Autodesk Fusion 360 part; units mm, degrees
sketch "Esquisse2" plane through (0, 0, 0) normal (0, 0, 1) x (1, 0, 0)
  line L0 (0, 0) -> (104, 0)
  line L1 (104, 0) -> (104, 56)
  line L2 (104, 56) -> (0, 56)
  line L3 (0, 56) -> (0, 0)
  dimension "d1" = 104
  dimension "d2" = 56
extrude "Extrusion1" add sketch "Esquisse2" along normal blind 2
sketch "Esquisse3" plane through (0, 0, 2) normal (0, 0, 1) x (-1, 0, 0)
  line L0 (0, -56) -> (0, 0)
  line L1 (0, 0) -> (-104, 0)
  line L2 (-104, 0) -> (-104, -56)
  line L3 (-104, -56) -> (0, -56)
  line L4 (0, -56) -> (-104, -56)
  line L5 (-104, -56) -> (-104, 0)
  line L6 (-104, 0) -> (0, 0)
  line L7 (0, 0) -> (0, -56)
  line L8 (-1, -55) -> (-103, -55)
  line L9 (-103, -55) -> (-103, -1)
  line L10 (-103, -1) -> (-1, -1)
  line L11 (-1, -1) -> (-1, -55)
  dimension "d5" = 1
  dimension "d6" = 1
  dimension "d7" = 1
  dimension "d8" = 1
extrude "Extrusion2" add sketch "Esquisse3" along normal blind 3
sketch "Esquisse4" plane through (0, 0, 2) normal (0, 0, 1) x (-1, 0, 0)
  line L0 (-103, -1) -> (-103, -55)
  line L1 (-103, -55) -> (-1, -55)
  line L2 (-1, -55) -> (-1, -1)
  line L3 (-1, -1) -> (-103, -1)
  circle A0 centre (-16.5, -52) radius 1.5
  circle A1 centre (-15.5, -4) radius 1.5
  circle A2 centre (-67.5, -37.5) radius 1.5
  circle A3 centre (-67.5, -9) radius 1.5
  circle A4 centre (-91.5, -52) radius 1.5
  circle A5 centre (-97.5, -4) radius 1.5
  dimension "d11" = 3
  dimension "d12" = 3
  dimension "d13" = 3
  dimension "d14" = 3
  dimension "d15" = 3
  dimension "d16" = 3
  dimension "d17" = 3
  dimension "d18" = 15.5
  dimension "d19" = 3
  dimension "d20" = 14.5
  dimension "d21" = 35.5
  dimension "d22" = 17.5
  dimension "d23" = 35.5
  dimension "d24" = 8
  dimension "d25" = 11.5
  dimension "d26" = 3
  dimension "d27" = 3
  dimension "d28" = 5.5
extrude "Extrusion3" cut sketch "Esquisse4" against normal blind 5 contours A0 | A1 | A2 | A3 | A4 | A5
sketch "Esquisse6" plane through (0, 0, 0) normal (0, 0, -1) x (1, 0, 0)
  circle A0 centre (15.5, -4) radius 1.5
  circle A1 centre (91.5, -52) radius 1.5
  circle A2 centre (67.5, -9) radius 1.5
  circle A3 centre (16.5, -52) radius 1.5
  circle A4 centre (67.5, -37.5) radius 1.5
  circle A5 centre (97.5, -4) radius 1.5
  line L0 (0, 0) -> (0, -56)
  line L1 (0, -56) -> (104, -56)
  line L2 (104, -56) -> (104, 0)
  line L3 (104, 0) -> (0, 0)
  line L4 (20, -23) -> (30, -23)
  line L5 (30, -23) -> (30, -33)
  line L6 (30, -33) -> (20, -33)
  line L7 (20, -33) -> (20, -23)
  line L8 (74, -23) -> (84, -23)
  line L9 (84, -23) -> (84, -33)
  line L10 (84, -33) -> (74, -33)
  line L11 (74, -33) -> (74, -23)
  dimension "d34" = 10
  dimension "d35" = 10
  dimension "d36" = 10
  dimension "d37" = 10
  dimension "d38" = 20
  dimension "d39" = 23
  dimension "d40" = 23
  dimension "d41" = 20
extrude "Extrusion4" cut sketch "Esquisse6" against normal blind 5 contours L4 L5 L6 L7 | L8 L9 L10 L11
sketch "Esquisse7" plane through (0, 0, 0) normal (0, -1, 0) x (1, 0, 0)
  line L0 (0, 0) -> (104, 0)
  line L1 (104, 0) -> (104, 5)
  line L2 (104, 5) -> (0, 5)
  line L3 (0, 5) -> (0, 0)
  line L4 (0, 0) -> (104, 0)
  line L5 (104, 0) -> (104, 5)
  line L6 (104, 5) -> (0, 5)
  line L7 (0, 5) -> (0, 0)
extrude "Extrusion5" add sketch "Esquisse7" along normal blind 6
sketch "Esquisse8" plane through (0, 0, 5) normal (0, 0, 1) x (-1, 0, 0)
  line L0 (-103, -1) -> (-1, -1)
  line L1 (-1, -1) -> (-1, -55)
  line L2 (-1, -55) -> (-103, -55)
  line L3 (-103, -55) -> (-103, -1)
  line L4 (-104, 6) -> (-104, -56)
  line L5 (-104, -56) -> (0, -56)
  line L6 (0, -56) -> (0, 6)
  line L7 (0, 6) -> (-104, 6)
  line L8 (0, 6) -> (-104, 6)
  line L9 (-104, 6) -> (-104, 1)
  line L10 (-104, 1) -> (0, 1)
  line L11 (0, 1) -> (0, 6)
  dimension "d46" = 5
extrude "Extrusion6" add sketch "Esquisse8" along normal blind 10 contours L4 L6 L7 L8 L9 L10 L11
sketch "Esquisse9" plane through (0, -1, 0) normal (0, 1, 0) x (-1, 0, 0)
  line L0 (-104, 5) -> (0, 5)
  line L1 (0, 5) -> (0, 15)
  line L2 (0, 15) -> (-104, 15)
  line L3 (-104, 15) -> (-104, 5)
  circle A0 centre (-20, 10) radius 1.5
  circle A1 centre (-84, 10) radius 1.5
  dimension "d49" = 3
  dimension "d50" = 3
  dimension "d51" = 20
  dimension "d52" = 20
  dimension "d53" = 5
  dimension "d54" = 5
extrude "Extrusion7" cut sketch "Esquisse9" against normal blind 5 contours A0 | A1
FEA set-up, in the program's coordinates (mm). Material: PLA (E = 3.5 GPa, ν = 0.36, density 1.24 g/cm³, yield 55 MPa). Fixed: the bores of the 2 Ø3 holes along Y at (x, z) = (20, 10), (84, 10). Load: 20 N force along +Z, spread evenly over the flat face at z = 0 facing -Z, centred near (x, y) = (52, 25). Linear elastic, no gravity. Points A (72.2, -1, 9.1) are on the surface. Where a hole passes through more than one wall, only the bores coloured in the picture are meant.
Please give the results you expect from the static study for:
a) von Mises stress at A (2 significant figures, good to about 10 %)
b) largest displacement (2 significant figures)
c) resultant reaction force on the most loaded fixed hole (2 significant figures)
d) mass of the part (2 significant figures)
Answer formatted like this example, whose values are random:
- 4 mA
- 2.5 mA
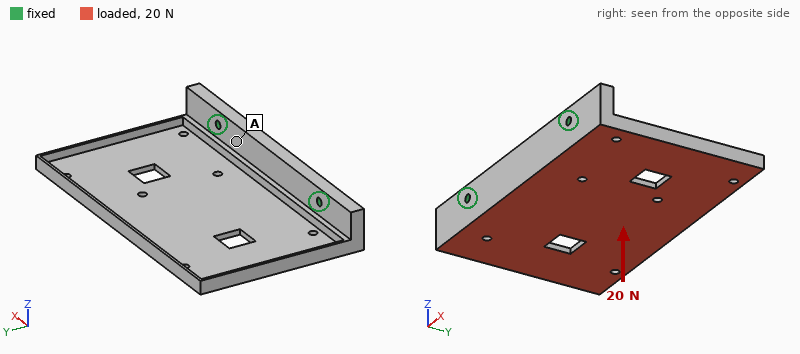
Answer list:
- 1.3 MPa
- 1.4 mm
- 10 N
- 25 g
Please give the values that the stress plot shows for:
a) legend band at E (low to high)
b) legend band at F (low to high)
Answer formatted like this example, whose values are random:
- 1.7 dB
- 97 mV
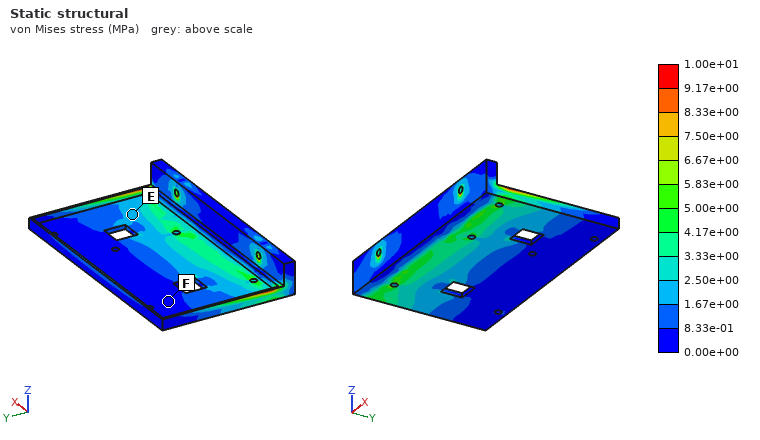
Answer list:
- 1.67e+00 to 2.50e+00 MPa
- 0.00e+00 to 8.33e-01 MPa
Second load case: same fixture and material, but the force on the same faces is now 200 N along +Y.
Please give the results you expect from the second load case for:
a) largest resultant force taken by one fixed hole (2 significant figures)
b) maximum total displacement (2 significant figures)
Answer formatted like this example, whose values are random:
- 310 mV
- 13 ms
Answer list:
- 100 N
- 1.0 mm
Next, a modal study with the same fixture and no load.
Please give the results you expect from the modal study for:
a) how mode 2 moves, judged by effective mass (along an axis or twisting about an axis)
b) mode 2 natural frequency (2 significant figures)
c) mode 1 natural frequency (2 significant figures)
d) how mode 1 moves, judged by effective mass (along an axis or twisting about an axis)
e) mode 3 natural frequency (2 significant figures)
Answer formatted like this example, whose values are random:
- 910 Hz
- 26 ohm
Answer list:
- twisting about Y
- 300 Hz
- 180 Hz
- along Z
- 650 Hz
